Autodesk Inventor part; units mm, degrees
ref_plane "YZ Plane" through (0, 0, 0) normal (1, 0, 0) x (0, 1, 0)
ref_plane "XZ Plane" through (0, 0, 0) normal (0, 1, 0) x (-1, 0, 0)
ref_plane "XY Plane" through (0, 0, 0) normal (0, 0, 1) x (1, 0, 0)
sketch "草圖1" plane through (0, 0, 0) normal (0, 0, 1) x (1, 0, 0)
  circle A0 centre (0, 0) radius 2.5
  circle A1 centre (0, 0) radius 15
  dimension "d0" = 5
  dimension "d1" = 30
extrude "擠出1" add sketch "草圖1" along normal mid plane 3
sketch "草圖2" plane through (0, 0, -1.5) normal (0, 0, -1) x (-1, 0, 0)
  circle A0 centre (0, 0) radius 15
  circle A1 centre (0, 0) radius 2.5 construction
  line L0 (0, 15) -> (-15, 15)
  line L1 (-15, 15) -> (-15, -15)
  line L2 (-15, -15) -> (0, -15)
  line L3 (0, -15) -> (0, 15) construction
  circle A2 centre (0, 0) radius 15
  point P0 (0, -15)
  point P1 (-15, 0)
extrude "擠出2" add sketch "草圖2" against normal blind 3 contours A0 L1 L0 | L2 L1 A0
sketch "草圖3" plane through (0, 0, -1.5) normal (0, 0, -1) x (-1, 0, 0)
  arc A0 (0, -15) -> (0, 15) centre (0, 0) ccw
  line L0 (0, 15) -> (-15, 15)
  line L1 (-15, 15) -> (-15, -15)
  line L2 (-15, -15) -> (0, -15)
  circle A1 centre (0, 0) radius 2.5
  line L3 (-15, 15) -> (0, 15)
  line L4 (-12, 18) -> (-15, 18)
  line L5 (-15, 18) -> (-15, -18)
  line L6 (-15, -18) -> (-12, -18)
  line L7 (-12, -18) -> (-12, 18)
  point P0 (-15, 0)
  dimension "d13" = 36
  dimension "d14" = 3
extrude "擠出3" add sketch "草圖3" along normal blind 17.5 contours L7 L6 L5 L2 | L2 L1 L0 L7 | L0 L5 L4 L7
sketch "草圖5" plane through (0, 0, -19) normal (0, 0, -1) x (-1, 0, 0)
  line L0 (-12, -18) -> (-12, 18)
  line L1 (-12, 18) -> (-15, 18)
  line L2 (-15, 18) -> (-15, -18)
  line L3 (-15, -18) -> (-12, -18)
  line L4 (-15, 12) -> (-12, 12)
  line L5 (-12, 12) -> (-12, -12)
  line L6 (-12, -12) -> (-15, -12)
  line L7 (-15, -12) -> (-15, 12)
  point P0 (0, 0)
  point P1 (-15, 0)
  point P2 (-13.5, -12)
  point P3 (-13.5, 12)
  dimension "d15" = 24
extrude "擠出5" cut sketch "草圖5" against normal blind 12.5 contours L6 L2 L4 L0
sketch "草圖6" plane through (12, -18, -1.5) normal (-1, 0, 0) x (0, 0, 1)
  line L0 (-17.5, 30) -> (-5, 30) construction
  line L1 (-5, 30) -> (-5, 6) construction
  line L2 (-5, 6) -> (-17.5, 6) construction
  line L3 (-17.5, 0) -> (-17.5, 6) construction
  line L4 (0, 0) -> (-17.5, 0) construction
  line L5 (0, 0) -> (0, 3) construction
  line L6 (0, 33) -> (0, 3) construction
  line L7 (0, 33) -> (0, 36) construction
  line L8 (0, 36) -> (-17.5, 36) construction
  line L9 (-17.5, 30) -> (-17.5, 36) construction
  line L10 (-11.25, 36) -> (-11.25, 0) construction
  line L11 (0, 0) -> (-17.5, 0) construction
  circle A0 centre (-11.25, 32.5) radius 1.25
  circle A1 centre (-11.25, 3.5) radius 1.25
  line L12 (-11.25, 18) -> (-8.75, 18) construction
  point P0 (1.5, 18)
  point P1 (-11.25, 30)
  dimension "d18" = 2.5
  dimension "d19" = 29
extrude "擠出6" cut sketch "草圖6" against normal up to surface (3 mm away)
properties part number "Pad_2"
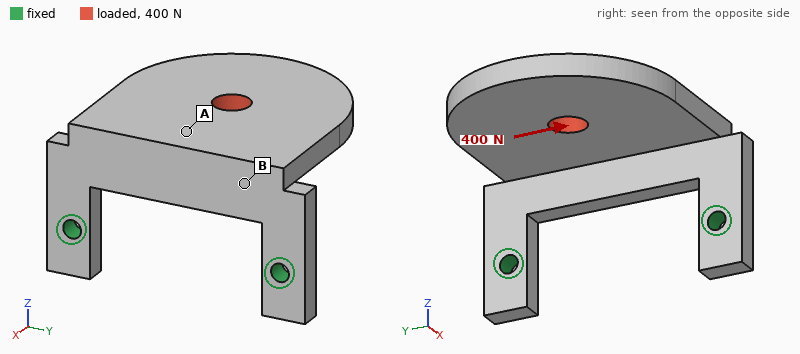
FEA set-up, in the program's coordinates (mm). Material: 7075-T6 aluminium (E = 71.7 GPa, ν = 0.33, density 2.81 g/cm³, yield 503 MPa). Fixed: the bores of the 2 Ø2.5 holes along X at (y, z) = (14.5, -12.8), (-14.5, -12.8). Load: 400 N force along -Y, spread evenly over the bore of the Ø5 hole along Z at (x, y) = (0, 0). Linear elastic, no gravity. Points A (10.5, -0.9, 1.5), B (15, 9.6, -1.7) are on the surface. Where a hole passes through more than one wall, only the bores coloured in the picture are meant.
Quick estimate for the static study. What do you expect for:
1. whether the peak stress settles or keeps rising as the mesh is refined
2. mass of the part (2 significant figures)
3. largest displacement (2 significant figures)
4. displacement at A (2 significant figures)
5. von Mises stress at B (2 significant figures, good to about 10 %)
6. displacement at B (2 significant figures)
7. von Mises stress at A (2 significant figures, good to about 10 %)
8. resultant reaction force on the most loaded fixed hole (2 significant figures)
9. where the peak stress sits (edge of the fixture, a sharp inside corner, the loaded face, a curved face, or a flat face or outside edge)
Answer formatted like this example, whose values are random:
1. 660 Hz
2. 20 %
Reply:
1. keeps rising
2. 9.3 g
3. 0.11 mm
4. 0.019 mm
5. 42 MPa
6. 0.027 mm
7. 17 MPa
8. 290 N
9. edge of the fixture
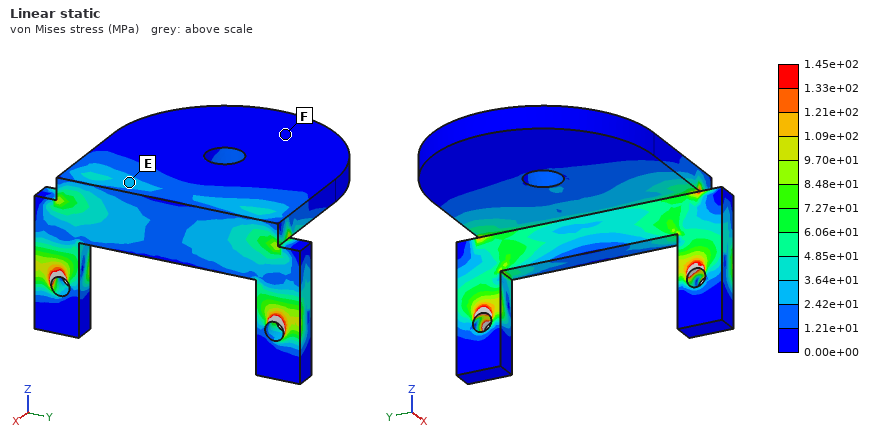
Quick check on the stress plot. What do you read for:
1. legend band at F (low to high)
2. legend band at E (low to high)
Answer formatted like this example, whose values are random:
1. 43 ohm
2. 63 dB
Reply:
1. 0.00e+00 to 1.21e+01 MPa
2. 2.42e+01 to 3.64e+01 MPa
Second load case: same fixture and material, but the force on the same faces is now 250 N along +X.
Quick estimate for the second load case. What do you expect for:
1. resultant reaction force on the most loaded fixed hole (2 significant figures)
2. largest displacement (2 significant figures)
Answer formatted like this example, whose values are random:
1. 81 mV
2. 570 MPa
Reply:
1. 130 N
2. 0.29 mm
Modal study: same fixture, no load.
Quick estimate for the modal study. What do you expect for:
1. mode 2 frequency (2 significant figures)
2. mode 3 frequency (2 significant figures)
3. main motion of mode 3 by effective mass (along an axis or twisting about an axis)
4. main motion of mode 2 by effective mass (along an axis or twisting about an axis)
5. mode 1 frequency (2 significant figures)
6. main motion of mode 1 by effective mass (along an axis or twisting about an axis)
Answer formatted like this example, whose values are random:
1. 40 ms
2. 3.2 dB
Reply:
1. 4400 Hz
2. 5500 Hz
3. along X
4. along Y
5. 1500 Hz
6. along Z
